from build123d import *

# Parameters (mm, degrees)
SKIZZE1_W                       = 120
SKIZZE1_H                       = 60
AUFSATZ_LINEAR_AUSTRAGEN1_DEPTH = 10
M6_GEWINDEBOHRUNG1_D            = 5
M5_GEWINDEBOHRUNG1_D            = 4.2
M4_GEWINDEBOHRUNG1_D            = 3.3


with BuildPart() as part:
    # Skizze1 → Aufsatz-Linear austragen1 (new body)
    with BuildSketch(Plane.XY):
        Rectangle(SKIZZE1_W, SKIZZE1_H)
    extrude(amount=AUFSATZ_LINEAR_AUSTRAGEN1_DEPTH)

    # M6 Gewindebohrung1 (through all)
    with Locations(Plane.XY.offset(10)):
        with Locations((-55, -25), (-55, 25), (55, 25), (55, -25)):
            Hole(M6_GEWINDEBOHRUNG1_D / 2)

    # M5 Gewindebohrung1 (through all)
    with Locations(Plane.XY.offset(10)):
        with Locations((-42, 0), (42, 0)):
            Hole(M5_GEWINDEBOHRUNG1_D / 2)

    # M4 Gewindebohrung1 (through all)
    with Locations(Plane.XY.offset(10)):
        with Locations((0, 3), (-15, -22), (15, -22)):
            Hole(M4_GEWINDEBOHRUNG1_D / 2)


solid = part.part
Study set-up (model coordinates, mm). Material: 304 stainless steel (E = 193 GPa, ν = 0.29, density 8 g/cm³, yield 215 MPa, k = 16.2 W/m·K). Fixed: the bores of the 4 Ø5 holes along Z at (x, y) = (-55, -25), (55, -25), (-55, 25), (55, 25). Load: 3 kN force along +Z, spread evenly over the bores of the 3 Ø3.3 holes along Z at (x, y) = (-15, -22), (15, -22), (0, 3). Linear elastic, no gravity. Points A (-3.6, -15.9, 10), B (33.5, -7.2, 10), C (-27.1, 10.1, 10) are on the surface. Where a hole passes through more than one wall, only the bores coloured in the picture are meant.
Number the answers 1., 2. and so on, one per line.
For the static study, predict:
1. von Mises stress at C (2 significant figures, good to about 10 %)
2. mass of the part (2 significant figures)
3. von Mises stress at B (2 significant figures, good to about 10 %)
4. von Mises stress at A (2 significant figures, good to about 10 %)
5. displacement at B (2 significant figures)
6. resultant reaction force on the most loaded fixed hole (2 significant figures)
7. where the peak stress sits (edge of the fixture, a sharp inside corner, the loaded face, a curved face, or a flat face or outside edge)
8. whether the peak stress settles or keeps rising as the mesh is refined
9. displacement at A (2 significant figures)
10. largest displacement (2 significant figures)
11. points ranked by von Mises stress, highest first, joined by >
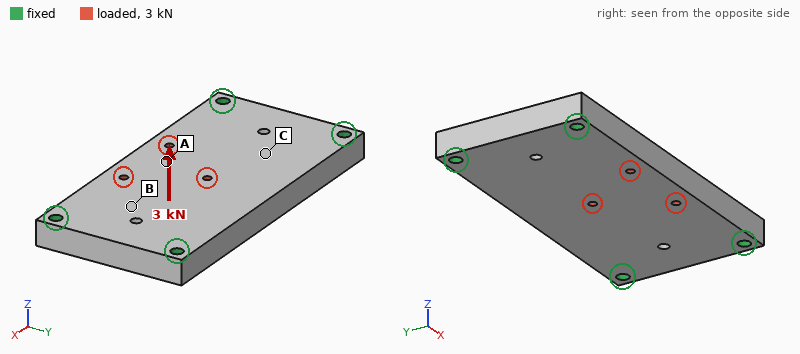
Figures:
1. 9.7 MPa
2. 570 g
3. 15 MPa
4. 33 MPa
5. 14 µm
6. 1.2 kN
7. edge of the fixture
8. keeps rising
9. 32 µm
10. 39 µm
11. A > B > C
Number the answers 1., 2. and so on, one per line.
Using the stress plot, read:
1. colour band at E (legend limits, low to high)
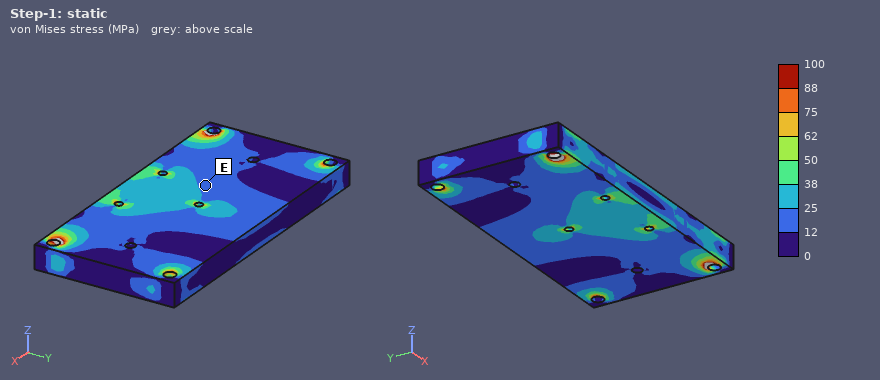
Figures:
1. 12 to 25 MPa
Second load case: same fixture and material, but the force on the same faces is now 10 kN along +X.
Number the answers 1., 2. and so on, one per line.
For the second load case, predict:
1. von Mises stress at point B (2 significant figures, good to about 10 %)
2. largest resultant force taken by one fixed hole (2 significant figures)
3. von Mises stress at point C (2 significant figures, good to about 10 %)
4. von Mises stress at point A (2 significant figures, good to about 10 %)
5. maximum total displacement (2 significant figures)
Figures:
1. 5.7 MPa
2. 2.9 kN
3. 7.1 MPa
4. 7.4 MPa
5. 4.3 µm
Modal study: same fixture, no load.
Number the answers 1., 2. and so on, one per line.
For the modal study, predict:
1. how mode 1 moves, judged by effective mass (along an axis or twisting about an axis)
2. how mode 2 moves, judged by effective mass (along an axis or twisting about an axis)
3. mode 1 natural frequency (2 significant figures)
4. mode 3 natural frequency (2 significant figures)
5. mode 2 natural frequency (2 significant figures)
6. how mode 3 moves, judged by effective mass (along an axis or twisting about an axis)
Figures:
1. along Z
2. twisting about X
3. 3400 Hz
4. 9000 Hz
5. 5900 Hz
6. twisting about Y
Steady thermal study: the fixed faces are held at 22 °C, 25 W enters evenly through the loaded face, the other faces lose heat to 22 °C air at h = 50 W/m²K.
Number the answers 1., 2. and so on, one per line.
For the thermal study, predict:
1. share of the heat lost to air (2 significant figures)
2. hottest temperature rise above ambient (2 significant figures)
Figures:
1. 63 %
2. 53 K
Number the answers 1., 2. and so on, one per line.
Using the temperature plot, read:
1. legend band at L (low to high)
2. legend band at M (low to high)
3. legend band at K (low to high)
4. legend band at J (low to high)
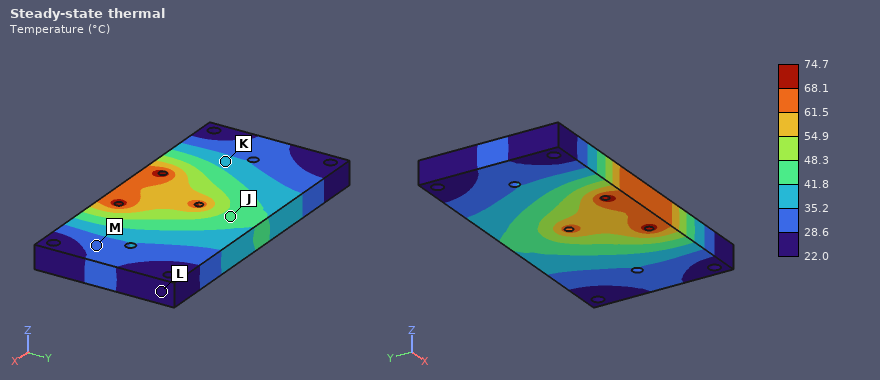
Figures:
1. 22.0 to 28.6 °C
2. 28.6 to 35.2 °C
3. 35.2 to 41.8 °C
4. 41.8 to 48.3 °C
